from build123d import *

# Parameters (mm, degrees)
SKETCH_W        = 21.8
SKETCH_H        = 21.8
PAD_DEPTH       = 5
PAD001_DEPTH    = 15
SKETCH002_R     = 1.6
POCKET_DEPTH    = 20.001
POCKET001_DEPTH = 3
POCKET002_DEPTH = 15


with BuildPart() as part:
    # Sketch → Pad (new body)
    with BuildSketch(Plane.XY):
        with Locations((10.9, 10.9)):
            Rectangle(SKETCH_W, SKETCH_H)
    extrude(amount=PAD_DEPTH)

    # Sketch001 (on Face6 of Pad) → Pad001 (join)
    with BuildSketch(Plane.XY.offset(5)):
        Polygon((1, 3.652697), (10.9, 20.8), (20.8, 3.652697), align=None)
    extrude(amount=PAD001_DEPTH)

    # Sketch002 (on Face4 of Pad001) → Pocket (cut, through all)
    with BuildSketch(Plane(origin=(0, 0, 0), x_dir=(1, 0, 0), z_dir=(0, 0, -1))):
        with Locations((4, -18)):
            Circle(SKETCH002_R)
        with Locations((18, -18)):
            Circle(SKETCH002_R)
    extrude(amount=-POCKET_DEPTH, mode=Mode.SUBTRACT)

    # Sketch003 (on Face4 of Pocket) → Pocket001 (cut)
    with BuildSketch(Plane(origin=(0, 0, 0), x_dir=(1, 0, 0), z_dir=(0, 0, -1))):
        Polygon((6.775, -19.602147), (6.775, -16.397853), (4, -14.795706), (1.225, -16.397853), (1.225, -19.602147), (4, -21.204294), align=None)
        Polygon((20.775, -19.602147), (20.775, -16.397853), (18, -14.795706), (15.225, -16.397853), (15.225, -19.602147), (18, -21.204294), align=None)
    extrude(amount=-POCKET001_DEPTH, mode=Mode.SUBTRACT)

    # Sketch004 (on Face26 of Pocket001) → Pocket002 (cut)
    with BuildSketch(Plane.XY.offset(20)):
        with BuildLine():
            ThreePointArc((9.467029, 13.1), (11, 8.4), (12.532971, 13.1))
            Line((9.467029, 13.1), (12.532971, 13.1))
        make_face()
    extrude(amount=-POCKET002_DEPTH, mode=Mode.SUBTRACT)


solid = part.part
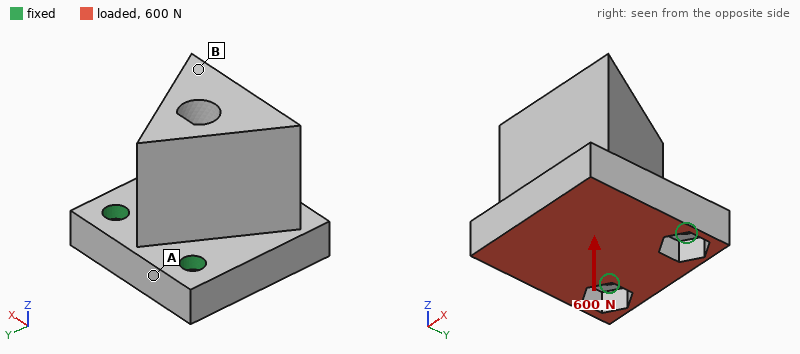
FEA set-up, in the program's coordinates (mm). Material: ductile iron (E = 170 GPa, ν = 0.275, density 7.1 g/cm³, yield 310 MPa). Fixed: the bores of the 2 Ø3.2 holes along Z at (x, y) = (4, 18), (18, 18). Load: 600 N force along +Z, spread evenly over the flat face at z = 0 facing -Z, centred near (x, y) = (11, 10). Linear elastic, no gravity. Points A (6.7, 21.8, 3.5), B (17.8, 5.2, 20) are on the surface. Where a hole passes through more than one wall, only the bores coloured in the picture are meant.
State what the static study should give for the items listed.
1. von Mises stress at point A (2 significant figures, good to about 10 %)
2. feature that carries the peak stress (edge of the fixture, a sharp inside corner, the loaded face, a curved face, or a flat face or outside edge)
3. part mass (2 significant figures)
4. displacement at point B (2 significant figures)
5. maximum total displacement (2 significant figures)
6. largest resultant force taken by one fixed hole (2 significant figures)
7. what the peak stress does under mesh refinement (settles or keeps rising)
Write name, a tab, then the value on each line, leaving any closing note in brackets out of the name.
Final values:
von Mises stress at point A	42 MPa
feature that carries the peak stress	edge of the fixture
part mass	31 g
displacement at point B	31 µm
maximum total displacement	33 µm
largest resultant force taken by one fixed hole	300 N
what the peak stress does under mesh refinement	keeps rising
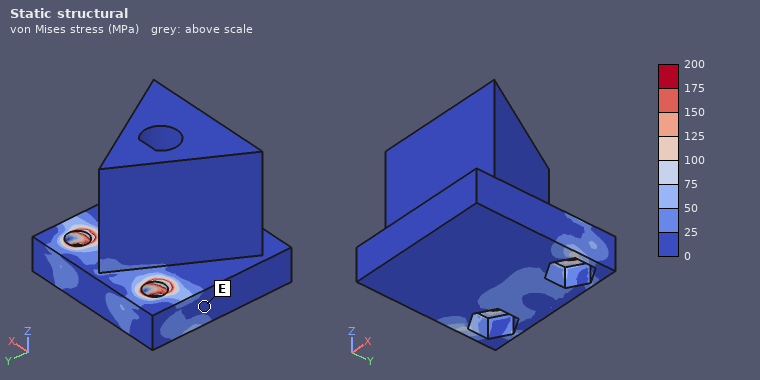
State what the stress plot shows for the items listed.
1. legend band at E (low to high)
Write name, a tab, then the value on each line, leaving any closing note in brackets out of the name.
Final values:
legend band at E	0 to 25 MPa
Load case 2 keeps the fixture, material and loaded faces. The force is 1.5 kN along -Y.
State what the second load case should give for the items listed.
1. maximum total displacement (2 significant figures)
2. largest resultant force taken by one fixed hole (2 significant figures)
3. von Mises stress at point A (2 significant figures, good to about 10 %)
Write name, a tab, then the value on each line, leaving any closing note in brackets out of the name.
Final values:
maximum total displacement	40 µm
largest resultant force taken by one fixed hole	770 N
von Mises stress at point A	55 MPa
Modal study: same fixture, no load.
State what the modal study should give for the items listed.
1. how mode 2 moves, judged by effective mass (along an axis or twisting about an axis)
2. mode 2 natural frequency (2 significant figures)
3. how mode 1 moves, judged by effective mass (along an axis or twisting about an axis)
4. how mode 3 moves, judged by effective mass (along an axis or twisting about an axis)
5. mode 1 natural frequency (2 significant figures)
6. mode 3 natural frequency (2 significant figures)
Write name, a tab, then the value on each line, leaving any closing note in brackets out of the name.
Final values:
how mode 2 moves, judged by effective mass	along X
mode 2 natural frequency	9700 Hz
how mode 1 moves, judged by effective mass	along Z
how mode 3 moves, judged by effective mass	along X
mode 1 natural frequency	4100 Hz
mode 3 natural frequency	21 kHz
